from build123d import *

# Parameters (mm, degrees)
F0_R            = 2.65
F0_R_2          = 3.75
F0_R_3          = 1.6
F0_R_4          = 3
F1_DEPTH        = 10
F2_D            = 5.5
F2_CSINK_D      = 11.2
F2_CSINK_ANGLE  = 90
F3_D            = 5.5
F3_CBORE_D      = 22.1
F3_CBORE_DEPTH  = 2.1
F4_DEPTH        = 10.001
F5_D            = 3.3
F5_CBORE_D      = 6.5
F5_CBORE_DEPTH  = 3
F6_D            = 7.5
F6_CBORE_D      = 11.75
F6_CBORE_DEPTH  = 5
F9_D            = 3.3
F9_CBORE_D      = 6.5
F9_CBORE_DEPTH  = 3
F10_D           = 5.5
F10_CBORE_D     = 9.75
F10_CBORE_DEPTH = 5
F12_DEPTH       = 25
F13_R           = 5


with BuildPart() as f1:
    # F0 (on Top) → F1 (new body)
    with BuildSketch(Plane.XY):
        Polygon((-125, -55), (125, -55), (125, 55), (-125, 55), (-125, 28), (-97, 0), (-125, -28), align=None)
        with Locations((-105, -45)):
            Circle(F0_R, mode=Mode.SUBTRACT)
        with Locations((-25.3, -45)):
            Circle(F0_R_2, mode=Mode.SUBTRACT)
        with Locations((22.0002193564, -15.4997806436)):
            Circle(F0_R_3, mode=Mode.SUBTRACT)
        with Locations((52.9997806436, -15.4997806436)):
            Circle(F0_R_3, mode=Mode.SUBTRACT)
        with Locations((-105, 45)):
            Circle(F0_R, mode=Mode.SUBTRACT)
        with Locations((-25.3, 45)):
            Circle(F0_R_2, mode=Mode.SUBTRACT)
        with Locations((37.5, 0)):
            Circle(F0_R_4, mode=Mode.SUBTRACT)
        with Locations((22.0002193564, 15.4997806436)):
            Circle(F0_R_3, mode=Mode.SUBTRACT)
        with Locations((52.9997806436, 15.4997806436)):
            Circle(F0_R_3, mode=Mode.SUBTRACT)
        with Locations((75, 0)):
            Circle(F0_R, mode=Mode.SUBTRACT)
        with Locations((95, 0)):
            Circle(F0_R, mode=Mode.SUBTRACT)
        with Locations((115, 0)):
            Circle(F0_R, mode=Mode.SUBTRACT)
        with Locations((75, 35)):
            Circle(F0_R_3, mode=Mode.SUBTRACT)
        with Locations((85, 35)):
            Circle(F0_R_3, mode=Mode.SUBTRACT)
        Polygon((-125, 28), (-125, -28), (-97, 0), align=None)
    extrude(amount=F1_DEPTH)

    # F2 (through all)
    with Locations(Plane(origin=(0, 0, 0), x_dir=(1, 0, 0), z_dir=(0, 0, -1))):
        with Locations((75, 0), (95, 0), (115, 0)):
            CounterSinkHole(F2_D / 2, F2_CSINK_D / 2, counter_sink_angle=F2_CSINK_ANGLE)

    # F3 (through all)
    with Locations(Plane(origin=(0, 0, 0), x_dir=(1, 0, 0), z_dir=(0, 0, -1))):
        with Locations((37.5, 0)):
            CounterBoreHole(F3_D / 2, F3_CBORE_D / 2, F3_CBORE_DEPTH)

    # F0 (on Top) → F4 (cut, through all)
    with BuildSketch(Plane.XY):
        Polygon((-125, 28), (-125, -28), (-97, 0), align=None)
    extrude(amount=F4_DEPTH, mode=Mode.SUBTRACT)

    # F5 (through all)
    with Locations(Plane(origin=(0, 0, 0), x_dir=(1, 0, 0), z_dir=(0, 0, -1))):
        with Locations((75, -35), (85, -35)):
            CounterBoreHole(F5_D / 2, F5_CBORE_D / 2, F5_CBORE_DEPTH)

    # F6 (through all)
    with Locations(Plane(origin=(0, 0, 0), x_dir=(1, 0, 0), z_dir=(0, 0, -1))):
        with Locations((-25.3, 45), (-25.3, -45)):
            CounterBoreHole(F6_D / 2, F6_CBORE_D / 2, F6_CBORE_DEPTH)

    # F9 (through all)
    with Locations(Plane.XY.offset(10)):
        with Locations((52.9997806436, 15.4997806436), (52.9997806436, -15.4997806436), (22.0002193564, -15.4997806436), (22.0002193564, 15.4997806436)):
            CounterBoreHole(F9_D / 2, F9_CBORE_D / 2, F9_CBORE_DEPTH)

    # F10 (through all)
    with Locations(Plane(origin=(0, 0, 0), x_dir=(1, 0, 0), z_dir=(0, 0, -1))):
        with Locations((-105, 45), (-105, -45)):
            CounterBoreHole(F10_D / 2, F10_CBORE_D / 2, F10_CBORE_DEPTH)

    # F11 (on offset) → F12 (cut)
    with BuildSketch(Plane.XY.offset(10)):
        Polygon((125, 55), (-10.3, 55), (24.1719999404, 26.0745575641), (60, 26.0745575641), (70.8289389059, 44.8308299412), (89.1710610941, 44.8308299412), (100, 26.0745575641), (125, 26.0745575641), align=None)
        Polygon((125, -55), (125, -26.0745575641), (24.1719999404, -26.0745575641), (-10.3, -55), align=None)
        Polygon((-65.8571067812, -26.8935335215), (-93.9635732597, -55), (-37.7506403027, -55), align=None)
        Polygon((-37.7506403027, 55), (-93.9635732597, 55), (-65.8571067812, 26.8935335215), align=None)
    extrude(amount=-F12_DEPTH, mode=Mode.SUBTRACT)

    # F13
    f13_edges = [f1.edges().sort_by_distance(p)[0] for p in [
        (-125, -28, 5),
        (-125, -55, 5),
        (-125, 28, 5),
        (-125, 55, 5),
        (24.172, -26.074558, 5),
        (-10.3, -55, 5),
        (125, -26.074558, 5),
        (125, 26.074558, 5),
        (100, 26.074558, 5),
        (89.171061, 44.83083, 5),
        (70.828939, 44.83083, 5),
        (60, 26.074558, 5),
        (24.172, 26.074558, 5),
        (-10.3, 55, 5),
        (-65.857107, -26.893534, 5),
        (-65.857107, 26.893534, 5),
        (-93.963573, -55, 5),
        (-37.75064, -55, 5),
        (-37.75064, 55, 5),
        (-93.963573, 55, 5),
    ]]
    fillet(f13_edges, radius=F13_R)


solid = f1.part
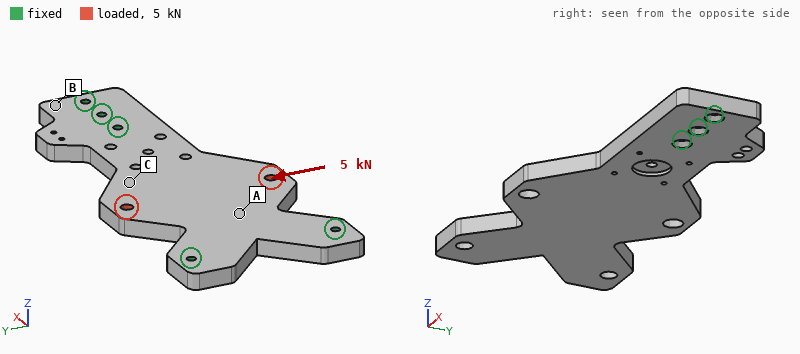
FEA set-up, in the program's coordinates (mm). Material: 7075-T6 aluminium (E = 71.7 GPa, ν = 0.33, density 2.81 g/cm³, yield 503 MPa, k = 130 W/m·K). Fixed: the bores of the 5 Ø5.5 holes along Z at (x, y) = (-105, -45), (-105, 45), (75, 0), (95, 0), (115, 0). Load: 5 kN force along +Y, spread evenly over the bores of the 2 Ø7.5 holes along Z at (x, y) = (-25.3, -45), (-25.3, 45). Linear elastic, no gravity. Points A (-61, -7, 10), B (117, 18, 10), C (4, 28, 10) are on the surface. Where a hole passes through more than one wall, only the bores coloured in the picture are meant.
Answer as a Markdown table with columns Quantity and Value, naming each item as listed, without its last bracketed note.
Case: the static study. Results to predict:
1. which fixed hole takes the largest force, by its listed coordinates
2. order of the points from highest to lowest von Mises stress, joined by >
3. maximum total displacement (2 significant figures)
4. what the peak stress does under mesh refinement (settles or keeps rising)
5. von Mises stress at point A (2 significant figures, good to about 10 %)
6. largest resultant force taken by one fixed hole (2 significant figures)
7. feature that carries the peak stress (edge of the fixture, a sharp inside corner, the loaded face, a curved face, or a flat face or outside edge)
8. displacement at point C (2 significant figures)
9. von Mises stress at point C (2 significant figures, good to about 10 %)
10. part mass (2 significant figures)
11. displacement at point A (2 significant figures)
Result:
| Quantity | Value |
|---|---|
| which fixed hole takes the largest force, by its listed coordinates | (75, 0) |
| order of the points from highest to lowest von Mises stress, joined by > | A > C > B |
| maximum total displacement | 63 µm |
| what the peak stress does under mesh refinement | keeps rising |
| von Mises stress at point A | 15 MPa |
| largest resultant force taken by one fixed hole | 2.5 kN |
| feature that carries the peak stress | edge of the fixture |
| displacement at point C | 32 µm |
| von Mises stress at point C | 8.1 MPa |
| part mass | 510 g |
| displacement at point A | 15 µm |
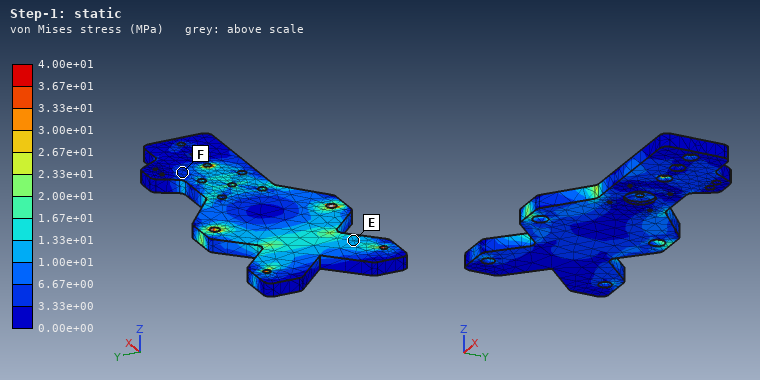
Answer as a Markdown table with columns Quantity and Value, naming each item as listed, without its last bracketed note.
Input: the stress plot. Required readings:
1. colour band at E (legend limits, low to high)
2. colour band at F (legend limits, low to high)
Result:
| Quantity | Value |
|---|---|
| colour band at E | 1.00e+01 to 1.33e+01 MPa |
| colour band at F | 3.33e+00 to 6.67e+00 MPa |
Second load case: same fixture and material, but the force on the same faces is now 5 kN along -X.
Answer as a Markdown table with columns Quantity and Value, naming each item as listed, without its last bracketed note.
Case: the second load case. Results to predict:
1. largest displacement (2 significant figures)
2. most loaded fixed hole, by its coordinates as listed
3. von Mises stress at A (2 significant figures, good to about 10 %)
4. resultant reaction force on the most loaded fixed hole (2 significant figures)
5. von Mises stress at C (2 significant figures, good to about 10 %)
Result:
| Quantity | Value |
|---|---|
| largest displacement | 18 µm |
| most loaded fixed hole, by its coordinates as listed | (75, 0) |
| von Mises stress at A | 4.5 MPa |
| resultant reaction force on the most loaded fixed hole | 1.8 kN |
| von Mises stress at C | 8.3 MPa |
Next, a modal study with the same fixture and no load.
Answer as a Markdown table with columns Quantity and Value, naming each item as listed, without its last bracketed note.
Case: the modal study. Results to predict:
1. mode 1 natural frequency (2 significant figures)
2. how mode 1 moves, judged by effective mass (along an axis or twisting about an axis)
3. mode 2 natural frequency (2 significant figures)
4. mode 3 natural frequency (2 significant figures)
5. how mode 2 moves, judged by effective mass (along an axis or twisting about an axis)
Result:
| Quantity | Value |
|---|---|
| mode 1 natural frequency | 1100 Hz |
| how mode 1 moves, judged by effective mass | along Z |
| mode 2 natural frequency | 1600 Hz |
| mode 3 natural frequency | 3100 Hz |
| how mode 2 moves, judged by effective mass | twisting about X |
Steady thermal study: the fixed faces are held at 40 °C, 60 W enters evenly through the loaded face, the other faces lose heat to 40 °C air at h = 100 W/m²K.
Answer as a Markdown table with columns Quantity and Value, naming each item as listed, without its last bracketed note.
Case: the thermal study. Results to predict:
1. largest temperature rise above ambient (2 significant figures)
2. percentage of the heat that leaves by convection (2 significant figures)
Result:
| Quantity | Value |
|---|---|
| largest temperature rise above ambient | 31 K |
| percentage of the heat that leaves by convection | 64 % |
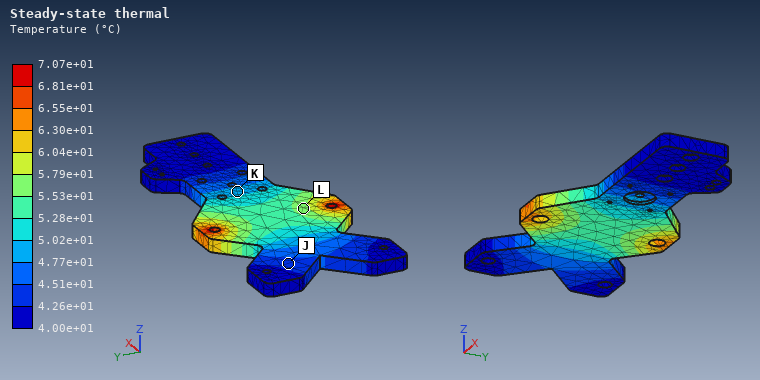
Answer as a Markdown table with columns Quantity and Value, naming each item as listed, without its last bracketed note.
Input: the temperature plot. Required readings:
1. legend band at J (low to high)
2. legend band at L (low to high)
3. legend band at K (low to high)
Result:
| Quantity | Value |
|---|---|
| legend band at J | 4.26e+01 to 4.51e+01 °C |
| legend band at L | 5.53e+01 to 5.79e+01 °C |
| legend band at K | 4.77e+01 to 5.02e+01 °C |
